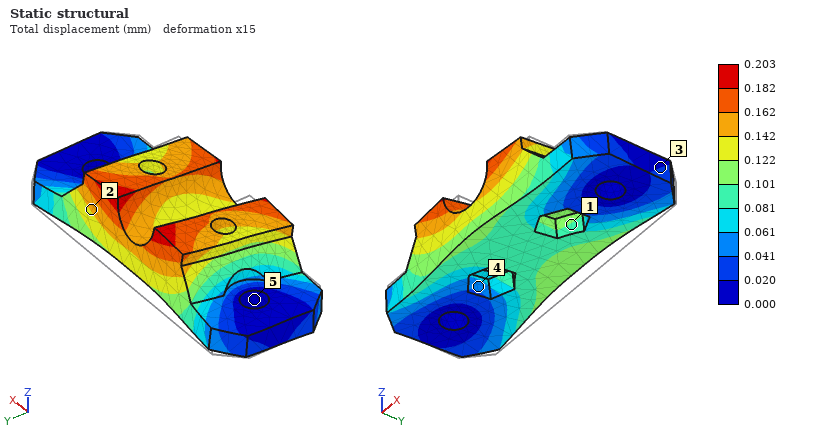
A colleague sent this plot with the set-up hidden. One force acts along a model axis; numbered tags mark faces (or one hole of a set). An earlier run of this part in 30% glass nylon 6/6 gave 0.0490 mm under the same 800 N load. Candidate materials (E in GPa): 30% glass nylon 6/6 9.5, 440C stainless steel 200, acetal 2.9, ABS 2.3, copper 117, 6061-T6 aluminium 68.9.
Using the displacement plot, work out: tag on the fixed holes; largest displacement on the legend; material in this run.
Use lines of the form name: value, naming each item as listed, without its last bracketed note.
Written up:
tag on the fixed holes: 5
largest displacement on the legend: 0.203 mm
material in this run: ABS
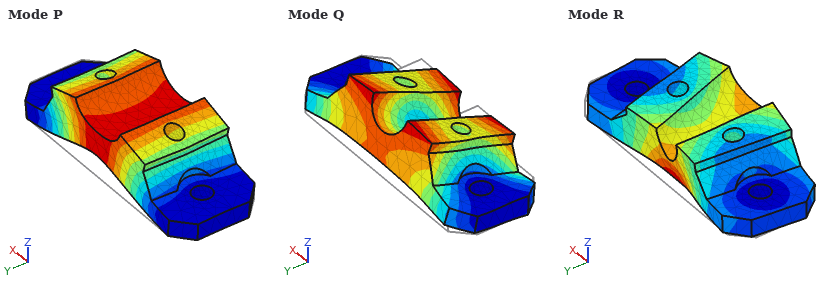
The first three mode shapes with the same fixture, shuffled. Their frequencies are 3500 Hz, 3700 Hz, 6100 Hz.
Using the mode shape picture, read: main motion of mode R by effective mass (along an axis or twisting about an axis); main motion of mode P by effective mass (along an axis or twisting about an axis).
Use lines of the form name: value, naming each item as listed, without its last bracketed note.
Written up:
main motion of mode R by effective mass: along Y
main motion of mode P by effective mass: along Z
